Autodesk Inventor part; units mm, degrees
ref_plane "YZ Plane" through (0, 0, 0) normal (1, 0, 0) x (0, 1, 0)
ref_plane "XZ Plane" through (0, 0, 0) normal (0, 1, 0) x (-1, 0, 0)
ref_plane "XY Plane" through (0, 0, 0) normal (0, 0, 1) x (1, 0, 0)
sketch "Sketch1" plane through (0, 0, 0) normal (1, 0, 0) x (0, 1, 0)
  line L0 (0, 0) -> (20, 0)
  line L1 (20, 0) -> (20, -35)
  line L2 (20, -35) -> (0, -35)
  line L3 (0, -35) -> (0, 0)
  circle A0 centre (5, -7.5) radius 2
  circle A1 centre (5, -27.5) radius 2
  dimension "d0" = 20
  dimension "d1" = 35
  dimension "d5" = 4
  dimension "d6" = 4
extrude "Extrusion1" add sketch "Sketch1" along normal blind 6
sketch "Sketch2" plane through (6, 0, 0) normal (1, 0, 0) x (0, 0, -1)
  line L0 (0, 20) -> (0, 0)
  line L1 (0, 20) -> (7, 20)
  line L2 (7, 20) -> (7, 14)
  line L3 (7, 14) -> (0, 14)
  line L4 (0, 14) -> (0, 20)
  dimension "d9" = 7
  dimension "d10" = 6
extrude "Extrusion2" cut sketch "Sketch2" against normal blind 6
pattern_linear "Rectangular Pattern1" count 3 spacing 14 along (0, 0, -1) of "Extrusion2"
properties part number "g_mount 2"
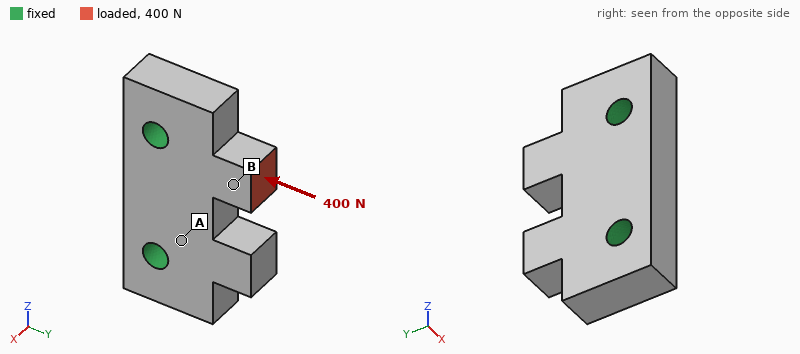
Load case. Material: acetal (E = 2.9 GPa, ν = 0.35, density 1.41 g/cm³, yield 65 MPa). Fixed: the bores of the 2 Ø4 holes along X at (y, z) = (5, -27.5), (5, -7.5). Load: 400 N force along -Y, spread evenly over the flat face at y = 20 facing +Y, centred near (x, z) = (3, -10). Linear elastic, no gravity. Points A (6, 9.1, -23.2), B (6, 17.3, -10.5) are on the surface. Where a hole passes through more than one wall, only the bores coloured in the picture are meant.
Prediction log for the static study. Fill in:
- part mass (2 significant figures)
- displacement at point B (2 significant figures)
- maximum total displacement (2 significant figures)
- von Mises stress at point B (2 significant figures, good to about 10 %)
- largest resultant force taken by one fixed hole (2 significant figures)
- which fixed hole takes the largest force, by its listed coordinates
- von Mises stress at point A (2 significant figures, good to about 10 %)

4.6 g
32 µm
45 µm
9.1 MPa
340 N
(5, -7.5)
1.8 MPa
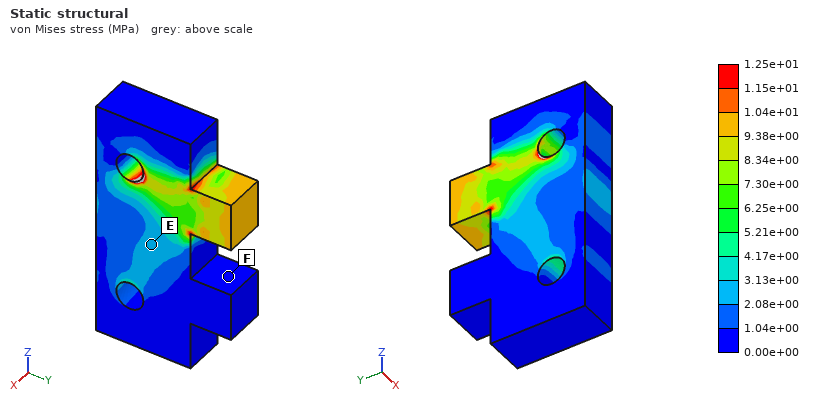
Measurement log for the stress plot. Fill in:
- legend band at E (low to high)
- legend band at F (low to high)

2.08e+00 to 3.13e+00 MPa
0.00e+00 to 1.04e+00 MPa
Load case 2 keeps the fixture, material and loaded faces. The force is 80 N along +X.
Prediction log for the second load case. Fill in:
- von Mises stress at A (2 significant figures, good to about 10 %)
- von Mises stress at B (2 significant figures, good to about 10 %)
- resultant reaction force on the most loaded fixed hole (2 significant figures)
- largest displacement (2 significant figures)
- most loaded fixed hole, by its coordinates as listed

2.9 MPa
5.3 MPa
72 N
0.15 mm
(5, -7.5)
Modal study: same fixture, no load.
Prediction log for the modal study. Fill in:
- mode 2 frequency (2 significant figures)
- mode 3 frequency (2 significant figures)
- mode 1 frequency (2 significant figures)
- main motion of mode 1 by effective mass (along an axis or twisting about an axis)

8700 Hz
13 kHz
6800 Hz
along X
